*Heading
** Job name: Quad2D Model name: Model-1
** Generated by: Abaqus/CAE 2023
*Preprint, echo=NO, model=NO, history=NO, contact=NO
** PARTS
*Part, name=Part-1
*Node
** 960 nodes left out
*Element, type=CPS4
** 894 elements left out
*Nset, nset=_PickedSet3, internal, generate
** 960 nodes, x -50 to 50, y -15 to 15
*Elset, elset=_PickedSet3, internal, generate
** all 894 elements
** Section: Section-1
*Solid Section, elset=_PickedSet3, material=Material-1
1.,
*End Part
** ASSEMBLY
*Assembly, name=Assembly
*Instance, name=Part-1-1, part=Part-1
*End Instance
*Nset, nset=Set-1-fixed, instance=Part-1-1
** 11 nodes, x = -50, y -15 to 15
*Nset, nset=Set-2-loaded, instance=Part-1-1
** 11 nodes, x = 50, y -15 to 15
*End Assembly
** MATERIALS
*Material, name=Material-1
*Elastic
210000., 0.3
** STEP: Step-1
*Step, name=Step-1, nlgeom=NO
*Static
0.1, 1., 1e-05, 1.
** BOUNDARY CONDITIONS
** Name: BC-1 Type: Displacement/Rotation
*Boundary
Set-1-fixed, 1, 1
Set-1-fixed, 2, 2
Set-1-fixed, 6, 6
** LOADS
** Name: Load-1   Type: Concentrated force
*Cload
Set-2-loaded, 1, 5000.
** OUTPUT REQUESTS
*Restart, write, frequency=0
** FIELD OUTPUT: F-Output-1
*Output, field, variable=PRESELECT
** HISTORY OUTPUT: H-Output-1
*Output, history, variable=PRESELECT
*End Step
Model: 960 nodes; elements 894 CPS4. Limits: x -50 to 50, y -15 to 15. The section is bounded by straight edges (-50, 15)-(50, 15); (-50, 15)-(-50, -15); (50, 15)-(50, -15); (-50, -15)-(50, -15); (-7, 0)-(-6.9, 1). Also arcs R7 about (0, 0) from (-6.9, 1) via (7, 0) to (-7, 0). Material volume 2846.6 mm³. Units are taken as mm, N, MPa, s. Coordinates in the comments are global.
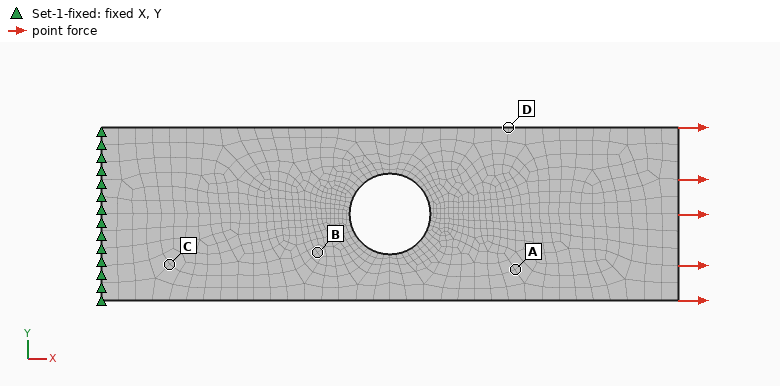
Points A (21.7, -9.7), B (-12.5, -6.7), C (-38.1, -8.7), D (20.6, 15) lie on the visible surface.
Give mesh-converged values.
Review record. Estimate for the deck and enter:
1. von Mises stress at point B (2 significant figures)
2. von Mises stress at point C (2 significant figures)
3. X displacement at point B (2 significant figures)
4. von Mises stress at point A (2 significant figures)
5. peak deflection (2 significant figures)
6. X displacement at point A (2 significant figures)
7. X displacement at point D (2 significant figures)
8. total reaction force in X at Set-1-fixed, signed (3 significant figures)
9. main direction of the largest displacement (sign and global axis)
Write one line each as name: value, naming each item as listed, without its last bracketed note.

von Mises stress at point B: 2100 MPa
von Mises stress at point C: 1800 MPa
X displacement at point B: 0.31 mm
von Mises stress at point A: 2000 MPa
peak deflection: 1.2 mm
X displacement at point A: 0.79 mm
X displacement at point D: 0.77 mm
total reaction force in X at Set-1-fixed, signed: -55000 N
main direction of the largest displacement: +X
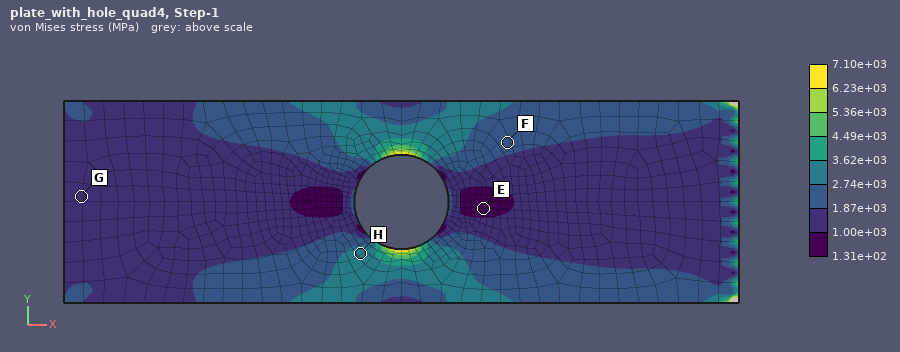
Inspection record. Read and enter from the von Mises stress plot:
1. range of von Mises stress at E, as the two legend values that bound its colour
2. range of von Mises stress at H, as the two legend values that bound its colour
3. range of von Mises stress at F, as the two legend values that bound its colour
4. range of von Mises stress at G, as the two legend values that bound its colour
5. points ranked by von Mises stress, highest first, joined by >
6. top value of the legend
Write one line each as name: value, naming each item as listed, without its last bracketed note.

range of von Mises stress at E, as the two legend values that bound its colour: 1.31e+02 to 1.00e+03 MPa
range of von Mises stress at H, as the two legend values that bound its colour: 2.74e+03 to 3.62e+03 MPa
range of von Mises stress at F, as the two legend values that bound its colour: 1.87e+03 to 2.74e+03 MPa
range of von Mises stress at G, as the two legend values that bound its colour: 1.00e+03 to 1.87e+03 MPa
points ranked by von Mises stress, highest first, joined by >: H > F > G > E
top value of the legend: 7.10e+03 MPa
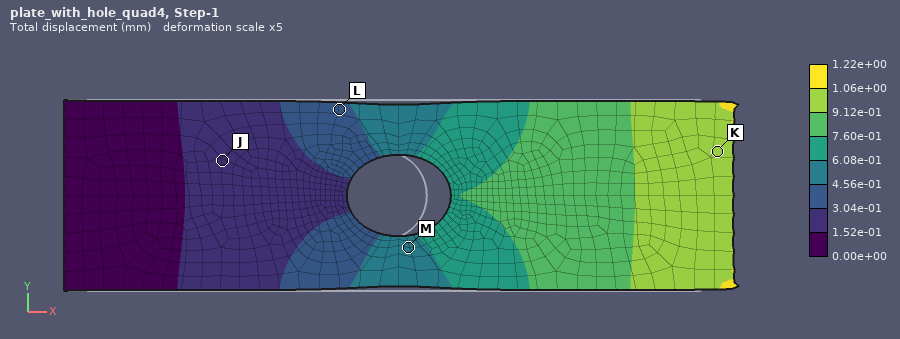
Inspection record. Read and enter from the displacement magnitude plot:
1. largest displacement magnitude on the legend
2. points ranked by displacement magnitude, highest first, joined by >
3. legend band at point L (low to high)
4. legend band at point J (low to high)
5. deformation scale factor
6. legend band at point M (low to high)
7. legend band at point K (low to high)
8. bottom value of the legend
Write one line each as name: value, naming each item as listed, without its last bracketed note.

largest displacement magnitude on the legend: 1.22e+00 mm
points ranked by displacement magnitude, highest first, joined by >: K > M > L > J
legend band at point L: 3.04e-01 to 4.56e-01 mm
legend band at point J: 1.52e-01 to 3.04e-01 mm
deformation scale factor: 5
legend band at point M: 4.56e-01 to 6.08e-01 mm
legend band at point K: 9.12e-01 to 1.06e+00 mm
bottom value of the legend: 0.00e+00 mm
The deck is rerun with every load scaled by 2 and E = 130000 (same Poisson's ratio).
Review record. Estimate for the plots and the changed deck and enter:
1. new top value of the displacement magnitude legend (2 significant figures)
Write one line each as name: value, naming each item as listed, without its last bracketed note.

new top value of the displacement magnitude legend: 3.9 mm
